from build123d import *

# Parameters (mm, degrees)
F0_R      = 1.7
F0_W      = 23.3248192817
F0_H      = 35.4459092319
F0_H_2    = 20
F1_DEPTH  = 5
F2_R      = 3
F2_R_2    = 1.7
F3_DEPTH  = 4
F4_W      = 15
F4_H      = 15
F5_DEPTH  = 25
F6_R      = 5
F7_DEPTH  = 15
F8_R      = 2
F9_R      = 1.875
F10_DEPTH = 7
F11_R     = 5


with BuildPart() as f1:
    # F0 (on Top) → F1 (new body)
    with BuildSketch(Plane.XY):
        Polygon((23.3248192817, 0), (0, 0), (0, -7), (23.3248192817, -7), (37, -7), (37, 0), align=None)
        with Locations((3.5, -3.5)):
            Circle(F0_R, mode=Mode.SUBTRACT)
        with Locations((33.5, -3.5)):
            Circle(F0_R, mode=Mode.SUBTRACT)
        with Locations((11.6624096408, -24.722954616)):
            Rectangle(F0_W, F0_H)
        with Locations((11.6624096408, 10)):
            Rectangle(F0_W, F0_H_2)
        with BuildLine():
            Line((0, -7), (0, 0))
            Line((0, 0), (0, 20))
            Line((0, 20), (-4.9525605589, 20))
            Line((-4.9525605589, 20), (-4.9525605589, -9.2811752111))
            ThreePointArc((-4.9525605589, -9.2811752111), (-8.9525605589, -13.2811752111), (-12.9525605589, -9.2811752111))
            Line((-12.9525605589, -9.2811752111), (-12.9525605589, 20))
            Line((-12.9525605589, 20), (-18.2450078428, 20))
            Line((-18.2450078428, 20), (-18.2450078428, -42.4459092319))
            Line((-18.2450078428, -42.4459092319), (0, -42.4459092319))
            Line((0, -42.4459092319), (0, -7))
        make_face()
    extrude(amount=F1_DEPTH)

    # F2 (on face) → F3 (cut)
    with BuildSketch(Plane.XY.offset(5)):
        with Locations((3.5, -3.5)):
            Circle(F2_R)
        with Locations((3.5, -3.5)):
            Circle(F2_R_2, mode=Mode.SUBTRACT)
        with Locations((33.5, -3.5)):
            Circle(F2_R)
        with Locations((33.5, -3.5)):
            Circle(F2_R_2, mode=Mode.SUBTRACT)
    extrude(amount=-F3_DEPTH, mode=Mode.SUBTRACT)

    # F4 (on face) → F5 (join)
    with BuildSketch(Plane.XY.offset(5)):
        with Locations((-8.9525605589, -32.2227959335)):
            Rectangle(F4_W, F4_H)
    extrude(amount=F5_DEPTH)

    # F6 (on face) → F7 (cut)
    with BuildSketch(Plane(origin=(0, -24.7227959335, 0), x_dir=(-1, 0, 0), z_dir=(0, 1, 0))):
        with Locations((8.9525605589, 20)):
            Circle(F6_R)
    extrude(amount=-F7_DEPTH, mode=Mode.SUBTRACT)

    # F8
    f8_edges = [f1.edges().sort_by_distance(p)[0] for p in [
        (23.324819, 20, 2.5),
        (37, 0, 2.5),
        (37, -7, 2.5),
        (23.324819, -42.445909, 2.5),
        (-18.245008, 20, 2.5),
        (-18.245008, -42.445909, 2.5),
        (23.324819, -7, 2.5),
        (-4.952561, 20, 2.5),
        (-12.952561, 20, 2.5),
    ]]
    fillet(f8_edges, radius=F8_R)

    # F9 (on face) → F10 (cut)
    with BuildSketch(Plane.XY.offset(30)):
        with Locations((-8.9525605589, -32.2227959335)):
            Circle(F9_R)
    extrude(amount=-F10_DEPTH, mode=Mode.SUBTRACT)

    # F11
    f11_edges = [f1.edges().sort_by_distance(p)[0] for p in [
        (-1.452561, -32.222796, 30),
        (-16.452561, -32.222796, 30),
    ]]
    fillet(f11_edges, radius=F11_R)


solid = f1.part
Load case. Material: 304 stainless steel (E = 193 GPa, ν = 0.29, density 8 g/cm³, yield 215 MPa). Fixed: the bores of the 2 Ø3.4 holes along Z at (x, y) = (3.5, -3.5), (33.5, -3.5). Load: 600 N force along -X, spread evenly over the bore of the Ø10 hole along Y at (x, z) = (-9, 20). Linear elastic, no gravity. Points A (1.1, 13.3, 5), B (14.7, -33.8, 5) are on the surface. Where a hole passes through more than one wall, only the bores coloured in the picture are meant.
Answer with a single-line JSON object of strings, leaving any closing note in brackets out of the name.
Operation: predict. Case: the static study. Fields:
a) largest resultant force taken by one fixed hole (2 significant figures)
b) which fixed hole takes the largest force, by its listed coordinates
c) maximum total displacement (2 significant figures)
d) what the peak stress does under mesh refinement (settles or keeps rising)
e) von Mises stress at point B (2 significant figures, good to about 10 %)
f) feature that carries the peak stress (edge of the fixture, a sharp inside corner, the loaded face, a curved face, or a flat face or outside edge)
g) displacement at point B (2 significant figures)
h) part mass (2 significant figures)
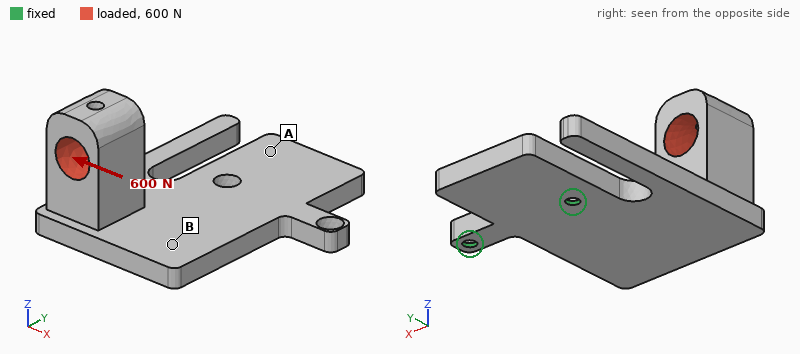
{"largest resultant force taken by one fixed hole": "1.1 kN", "which fixed hole takes the largest force, by its listed coordinates": "(33.5, -3.5)", "maximum total displacement": "0.15 mm", "what the peak stress does under mesh refinement": "keeps rising", "von Mises stress at point B": "36 MPa", "feature that carries the peak stress": "edge of the fixture", "displacement at point B": "0.039 mm", "part mass": "130 g"}
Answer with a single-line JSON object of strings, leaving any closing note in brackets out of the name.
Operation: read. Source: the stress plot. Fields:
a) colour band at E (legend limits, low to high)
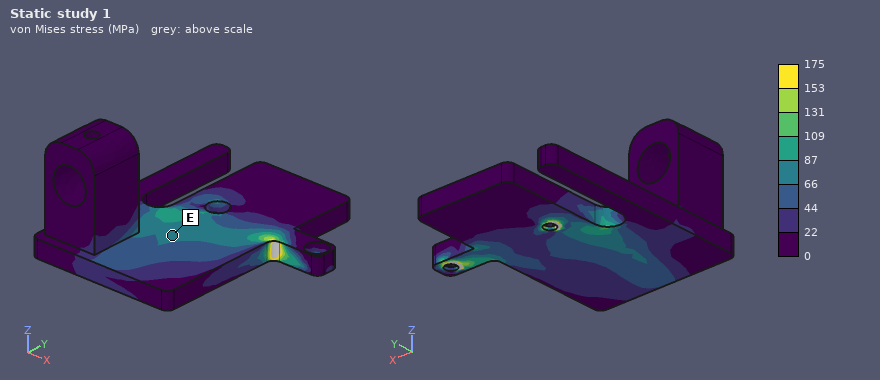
{"colour band at E": "66 to 87 MPa"}
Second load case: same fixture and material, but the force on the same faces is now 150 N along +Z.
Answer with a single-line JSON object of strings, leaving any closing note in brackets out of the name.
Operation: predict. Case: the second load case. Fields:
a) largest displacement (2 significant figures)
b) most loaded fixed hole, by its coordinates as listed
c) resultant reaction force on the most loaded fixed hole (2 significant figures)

{"largest displacement": "0.20 mm", "most loaded fixed hole, by its coordinates as listed": "(3.5, -3.5)", "resultant reaction force on the most loaded fixed hole": "230 N"}
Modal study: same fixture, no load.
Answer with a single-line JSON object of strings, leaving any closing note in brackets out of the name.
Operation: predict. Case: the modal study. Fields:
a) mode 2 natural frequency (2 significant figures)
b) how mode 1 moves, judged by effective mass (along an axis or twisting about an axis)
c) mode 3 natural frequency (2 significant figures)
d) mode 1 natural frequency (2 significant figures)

{"mode 2 natural frequency": "1800 Hz", "how mode 1 moves, judged by effective mass": "along Z", "mode 3 natural frequency": "2500 Hz", "mode 1 natural frequency": "590 Hz"}
